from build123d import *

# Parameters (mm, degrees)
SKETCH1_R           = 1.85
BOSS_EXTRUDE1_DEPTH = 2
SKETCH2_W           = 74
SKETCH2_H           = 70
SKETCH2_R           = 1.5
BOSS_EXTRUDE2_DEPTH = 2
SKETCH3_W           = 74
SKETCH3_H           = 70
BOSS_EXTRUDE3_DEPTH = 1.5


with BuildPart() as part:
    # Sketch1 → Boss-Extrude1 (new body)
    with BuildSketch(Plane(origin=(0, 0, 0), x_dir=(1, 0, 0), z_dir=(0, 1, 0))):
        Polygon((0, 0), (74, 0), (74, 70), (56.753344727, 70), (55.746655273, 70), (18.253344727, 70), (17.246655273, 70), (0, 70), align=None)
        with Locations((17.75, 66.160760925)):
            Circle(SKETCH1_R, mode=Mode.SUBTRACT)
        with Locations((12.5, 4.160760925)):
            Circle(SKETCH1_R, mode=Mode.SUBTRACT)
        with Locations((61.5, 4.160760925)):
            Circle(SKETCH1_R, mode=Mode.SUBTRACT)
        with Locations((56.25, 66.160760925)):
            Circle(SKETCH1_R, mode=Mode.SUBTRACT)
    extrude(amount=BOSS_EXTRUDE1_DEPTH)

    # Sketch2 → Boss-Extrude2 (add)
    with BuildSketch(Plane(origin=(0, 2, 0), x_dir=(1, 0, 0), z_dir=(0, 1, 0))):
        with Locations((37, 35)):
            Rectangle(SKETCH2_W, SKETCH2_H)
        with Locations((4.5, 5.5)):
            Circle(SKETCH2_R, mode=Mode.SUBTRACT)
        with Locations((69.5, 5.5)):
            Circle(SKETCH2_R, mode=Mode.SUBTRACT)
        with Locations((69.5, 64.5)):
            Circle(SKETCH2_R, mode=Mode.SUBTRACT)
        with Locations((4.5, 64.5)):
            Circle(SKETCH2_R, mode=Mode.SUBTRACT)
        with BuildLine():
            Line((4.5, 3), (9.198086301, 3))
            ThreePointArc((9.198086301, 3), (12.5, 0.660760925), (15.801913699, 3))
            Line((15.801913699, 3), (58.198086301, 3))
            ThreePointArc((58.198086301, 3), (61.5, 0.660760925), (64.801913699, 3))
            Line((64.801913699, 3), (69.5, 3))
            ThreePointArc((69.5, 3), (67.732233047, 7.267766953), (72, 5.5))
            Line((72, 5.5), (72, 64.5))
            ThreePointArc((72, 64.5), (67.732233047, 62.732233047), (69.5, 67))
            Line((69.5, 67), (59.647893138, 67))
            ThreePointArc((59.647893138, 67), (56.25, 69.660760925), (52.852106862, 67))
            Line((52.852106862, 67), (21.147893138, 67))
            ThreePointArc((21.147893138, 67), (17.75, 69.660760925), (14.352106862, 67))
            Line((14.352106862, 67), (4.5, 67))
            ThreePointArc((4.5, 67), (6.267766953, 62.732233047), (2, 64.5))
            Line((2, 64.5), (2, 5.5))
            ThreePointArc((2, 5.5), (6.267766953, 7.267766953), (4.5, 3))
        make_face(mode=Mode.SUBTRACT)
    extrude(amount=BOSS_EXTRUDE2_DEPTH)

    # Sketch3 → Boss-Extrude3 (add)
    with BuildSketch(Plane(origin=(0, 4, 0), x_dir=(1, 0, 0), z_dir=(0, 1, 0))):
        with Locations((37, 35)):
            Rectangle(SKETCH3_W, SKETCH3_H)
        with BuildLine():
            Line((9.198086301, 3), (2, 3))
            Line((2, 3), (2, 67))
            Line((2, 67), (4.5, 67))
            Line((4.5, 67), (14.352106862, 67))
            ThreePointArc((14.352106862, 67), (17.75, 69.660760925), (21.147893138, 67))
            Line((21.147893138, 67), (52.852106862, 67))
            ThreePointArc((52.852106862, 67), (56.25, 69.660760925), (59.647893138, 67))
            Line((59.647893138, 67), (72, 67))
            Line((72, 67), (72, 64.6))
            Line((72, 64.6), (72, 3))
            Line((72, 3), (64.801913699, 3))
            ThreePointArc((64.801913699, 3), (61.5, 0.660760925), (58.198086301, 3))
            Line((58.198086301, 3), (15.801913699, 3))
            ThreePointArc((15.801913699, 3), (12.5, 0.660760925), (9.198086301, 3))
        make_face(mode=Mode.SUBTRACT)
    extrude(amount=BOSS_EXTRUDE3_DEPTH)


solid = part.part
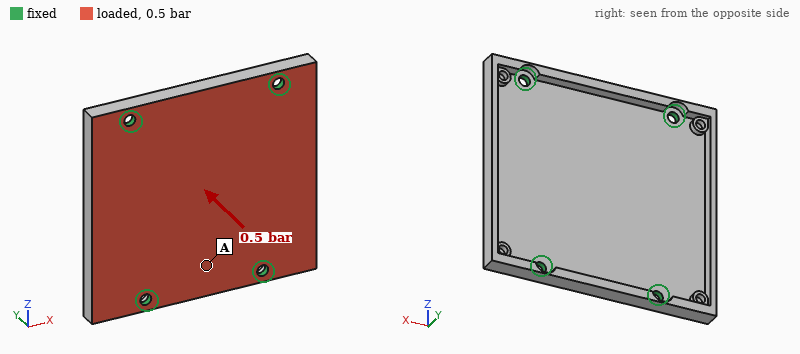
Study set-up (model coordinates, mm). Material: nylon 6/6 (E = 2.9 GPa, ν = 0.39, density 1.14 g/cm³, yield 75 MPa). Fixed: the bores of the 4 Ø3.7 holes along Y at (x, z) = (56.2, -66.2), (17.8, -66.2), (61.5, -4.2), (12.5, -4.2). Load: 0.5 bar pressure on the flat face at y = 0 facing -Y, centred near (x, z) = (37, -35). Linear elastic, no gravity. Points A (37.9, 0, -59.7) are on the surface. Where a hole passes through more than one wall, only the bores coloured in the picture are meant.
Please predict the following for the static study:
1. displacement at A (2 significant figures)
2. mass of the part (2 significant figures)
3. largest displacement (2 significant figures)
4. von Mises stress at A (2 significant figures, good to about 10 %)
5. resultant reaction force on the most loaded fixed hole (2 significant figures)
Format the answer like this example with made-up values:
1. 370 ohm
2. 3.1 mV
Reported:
1. 0.30 mm
2. 14 g
3. 1.1 mm
4. 4.1 MPa
5. 67 N
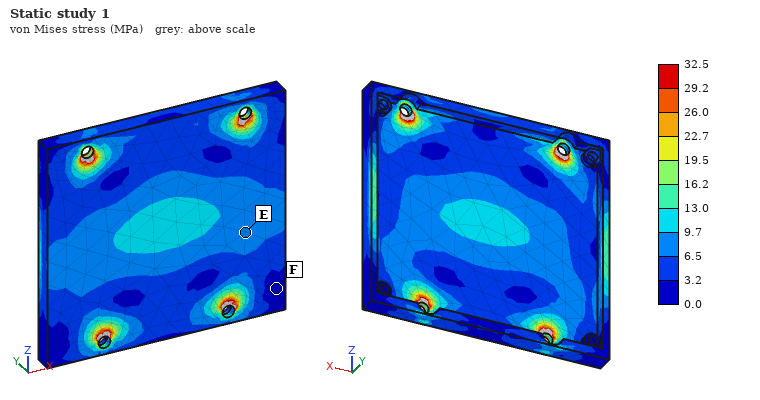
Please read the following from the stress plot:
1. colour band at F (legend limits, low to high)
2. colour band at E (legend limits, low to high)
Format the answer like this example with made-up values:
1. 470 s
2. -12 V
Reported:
1. 0.0 to 3.2 MPa
2. 6.5 to 9.7 MPa
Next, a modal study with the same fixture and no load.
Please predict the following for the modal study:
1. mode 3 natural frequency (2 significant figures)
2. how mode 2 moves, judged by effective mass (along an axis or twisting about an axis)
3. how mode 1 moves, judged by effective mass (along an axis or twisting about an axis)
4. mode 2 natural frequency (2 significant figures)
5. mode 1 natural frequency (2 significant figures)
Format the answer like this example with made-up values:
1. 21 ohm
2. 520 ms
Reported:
1. 1200 Hz
2. twisting about Z
3. along Y
4. 1100 Hz
5. 870 Hz
